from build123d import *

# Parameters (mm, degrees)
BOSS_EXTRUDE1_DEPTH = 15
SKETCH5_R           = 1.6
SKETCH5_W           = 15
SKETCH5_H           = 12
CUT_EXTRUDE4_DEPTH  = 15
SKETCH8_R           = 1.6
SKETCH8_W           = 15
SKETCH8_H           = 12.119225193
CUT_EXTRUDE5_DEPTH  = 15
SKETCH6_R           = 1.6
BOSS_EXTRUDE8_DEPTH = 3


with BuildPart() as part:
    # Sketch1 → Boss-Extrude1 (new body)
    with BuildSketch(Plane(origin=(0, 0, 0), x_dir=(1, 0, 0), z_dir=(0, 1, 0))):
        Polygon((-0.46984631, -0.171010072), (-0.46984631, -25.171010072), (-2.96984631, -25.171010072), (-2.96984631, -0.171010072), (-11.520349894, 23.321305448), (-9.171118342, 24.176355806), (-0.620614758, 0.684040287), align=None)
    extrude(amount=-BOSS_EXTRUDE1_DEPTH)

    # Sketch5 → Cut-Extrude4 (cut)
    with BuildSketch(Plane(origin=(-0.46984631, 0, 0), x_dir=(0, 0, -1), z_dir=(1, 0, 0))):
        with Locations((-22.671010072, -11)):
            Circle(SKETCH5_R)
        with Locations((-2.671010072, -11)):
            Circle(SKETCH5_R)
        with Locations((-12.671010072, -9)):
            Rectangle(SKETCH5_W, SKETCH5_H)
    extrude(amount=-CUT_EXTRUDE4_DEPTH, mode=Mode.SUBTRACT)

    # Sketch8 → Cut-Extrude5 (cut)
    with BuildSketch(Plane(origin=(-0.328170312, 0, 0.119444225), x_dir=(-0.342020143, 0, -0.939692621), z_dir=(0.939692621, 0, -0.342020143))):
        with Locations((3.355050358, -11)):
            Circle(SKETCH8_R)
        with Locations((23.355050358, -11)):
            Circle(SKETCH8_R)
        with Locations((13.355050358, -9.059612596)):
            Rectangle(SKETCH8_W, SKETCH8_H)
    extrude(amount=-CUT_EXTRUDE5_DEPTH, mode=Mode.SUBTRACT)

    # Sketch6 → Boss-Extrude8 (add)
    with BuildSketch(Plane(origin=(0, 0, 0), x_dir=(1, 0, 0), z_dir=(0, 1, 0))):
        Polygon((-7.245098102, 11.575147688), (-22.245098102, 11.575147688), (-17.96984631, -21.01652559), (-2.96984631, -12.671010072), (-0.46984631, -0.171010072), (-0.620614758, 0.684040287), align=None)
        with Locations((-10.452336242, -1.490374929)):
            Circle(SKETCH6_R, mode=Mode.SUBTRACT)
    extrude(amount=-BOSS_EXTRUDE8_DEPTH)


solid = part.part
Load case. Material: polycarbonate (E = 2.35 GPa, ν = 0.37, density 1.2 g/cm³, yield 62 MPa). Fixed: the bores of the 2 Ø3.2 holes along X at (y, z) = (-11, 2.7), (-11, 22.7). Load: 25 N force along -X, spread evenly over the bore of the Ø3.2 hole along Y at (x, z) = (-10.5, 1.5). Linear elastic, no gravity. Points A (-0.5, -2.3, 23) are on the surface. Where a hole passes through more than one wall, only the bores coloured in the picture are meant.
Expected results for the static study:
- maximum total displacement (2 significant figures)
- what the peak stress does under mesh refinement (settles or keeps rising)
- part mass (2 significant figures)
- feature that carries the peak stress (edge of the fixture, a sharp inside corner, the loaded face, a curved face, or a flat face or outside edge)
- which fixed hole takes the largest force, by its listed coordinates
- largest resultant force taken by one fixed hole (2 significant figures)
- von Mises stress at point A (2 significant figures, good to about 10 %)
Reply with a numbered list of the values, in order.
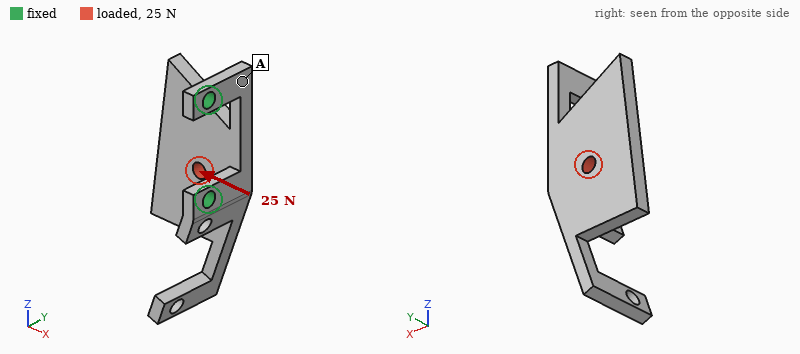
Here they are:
1. 0.63 mm
2. keeps rising
3. 2.8 g
4. edge of the fixture
5. (-11, 2.7)
6. 24 N
7. 2.7 MPa
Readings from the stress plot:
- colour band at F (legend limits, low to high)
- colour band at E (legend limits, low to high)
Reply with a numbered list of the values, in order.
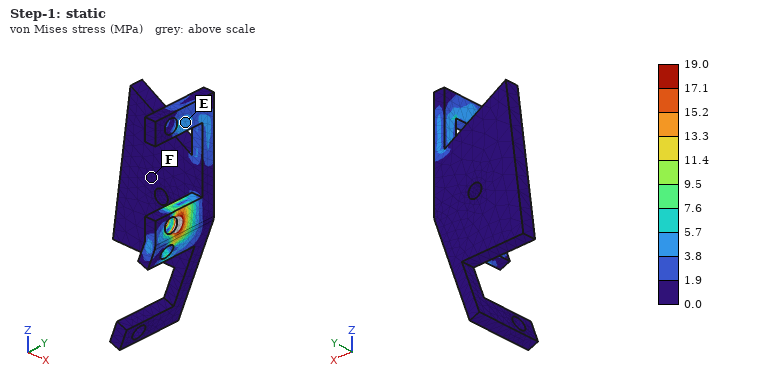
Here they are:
1. 0.0 to 1.9 MPa
2. 3.8 to 5.7 MPa
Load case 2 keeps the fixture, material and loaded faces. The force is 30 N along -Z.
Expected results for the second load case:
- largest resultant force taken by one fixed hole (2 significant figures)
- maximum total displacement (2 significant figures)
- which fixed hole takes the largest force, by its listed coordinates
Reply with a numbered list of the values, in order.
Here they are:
1. 21 N
2. 0.66 mm
3. (-11, 2.7)
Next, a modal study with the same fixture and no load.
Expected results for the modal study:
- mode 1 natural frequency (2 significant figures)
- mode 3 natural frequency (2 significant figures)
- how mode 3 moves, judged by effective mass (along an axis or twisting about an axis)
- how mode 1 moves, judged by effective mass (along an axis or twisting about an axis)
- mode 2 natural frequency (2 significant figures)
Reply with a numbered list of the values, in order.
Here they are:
1. 570 Hz
2. 930 Hz
3. twisting about X
4. along Y
5. 740 Hz
